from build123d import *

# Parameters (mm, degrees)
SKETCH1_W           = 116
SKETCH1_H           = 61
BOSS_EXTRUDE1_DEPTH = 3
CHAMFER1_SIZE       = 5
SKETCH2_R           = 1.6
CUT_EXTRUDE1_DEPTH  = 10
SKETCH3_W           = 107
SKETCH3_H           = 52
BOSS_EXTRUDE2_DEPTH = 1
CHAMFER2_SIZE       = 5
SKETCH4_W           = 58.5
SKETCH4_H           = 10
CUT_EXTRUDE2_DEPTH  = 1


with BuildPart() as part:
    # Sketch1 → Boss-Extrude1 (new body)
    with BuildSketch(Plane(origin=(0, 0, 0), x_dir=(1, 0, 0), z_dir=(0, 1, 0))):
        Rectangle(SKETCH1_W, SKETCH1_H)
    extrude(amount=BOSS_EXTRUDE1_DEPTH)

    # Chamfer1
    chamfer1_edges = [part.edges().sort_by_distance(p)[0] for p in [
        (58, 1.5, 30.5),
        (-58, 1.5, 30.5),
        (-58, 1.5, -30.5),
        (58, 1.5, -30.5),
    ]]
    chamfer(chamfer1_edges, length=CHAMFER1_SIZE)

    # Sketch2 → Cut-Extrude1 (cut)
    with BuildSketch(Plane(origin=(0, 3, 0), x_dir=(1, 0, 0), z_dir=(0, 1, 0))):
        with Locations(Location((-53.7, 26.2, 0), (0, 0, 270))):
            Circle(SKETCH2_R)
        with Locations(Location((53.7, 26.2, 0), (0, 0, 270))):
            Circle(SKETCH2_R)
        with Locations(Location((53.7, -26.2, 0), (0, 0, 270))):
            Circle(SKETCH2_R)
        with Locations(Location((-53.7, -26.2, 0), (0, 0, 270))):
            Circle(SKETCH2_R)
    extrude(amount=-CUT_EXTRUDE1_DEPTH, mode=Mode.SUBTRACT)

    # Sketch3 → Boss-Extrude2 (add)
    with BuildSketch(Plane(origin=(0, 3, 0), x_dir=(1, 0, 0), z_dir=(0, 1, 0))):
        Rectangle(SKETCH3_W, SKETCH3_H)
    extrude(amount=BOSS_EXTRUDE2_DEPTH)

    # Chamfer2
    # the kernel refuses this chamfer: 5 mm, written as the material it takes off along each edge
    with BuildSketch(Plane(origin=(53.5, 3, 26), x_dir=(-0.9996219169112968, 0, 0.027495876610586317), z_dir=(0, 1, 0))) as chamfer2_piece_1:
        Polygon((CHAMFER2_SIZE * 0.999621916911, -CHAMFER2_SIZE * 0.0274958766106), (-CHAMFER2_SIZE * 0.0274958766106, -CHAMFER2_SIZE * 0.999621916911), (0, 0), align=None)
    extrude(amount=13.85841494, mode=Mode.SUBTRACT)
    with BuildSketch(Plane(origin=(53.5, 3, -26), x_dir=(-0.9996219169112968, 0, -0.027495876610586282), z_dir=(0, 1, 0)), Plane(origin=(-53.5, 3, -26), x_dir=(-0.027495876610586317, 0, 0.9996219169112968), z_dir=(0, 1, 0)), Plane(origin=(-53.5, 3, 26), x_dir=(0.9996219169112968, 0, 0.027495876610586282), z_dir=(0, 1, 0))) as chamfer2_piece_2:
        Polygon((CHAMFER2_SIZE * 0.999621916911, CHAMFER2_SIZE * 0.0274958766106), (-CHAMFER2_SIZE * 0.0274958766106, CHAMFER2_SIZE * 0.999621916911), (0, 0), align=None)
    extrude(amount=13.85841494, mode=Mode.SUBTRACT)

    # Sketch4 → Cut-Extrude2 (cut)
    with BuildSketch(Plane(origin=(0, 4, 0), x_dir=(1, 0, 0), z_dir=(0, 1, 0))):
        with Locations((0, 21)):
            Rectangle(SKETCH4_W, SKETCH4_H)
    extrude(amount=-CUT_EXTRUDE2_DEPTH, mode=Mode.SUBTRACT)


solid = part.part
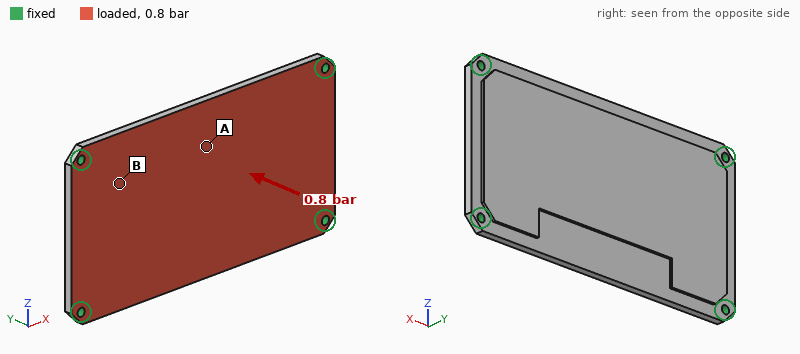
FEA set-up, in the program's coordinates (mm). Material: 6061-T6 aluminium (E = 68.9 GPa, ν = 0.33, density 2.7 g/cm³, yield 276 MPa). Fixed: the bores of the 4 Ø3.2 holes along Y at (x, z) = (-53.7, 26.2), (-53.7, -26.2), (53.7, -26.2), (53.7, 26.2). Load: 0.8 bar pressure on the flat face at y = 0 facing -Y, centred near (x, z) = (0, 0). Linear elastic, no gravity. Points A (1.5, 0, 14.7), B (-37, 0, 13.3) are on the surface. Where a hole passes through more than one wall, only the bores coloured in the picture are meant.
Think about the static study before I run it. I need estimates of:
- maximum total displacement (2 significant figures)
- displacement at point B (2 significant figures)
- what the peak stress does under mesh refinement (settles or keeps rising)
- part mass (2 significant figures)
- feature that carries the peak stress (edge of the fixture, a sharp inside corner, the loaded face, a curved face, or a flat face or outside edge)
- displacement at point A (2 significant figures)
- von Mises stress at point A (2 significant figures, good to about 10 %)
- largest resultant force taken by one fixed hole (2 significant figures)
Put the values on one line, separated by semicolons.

0.18 mm; 0.066 mm; keeps rising; 70 g; edge of the fixture; 0.16 mm; 20 MPa; 210 N
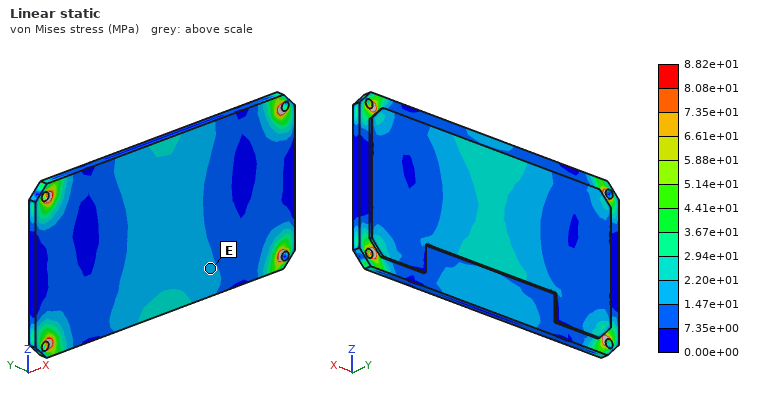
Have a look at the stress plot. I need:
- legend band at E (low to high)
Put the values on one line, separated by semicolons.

1.47e+01 to 2.20e+01 MPa
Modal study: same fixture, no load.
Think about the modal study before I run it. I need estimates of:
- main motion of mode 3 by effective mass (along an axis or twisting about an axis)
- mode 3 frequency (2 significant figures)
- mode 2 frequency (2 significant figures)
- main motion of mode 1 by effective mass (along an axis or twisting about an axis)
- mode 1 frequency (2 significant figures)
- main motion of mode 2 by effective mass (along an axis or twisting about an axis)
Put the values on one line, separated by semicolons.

twisting about Z; 3600 Hz; 2500 Hz; along Y; 1300 Hz; twisting about X
